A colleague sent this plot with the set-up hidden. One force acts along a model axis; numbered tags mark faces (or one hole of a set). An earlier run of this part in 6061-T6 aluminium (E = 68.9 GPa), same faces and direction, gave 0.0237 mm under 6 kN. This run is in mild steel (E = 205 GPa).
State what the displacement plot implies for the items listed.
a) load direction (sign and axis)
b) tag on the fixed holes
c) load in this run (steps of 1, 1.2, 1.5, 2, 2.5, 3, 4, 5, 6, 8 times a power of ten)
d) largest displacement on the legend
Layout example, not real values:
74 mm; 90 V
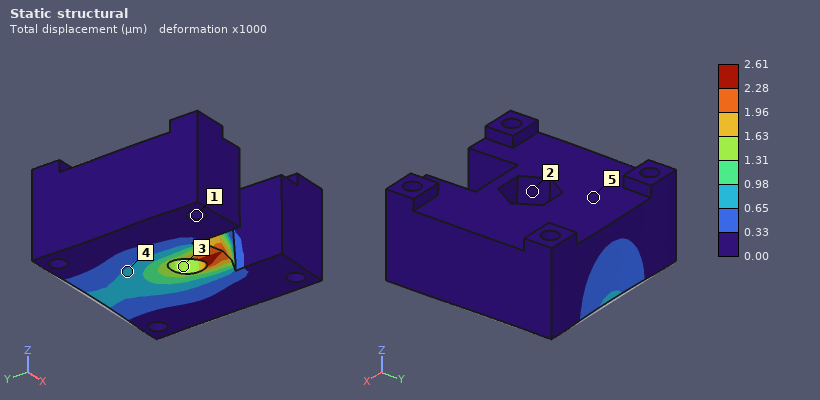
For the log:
-Y; 1; 2 kN; 2.61 µm
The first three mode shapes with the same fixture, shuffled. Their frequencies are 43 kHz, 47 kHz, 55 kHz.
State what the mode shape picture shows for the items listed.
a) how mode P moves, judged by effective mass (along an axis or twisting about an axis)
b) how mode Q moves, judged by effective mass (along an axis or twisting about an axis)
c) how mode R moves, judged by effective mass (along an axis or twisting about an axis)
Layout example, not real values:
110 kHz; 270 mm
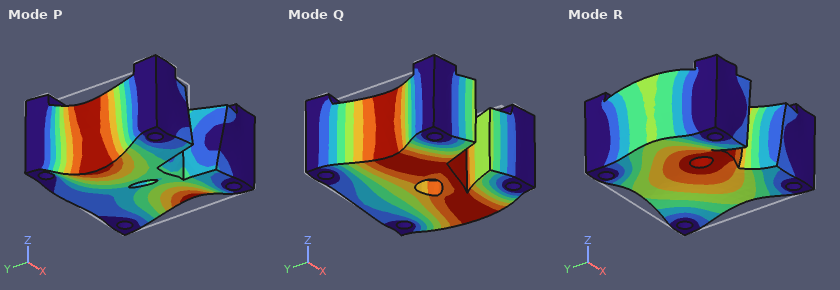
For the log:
twisting about Y; along X; along Z
